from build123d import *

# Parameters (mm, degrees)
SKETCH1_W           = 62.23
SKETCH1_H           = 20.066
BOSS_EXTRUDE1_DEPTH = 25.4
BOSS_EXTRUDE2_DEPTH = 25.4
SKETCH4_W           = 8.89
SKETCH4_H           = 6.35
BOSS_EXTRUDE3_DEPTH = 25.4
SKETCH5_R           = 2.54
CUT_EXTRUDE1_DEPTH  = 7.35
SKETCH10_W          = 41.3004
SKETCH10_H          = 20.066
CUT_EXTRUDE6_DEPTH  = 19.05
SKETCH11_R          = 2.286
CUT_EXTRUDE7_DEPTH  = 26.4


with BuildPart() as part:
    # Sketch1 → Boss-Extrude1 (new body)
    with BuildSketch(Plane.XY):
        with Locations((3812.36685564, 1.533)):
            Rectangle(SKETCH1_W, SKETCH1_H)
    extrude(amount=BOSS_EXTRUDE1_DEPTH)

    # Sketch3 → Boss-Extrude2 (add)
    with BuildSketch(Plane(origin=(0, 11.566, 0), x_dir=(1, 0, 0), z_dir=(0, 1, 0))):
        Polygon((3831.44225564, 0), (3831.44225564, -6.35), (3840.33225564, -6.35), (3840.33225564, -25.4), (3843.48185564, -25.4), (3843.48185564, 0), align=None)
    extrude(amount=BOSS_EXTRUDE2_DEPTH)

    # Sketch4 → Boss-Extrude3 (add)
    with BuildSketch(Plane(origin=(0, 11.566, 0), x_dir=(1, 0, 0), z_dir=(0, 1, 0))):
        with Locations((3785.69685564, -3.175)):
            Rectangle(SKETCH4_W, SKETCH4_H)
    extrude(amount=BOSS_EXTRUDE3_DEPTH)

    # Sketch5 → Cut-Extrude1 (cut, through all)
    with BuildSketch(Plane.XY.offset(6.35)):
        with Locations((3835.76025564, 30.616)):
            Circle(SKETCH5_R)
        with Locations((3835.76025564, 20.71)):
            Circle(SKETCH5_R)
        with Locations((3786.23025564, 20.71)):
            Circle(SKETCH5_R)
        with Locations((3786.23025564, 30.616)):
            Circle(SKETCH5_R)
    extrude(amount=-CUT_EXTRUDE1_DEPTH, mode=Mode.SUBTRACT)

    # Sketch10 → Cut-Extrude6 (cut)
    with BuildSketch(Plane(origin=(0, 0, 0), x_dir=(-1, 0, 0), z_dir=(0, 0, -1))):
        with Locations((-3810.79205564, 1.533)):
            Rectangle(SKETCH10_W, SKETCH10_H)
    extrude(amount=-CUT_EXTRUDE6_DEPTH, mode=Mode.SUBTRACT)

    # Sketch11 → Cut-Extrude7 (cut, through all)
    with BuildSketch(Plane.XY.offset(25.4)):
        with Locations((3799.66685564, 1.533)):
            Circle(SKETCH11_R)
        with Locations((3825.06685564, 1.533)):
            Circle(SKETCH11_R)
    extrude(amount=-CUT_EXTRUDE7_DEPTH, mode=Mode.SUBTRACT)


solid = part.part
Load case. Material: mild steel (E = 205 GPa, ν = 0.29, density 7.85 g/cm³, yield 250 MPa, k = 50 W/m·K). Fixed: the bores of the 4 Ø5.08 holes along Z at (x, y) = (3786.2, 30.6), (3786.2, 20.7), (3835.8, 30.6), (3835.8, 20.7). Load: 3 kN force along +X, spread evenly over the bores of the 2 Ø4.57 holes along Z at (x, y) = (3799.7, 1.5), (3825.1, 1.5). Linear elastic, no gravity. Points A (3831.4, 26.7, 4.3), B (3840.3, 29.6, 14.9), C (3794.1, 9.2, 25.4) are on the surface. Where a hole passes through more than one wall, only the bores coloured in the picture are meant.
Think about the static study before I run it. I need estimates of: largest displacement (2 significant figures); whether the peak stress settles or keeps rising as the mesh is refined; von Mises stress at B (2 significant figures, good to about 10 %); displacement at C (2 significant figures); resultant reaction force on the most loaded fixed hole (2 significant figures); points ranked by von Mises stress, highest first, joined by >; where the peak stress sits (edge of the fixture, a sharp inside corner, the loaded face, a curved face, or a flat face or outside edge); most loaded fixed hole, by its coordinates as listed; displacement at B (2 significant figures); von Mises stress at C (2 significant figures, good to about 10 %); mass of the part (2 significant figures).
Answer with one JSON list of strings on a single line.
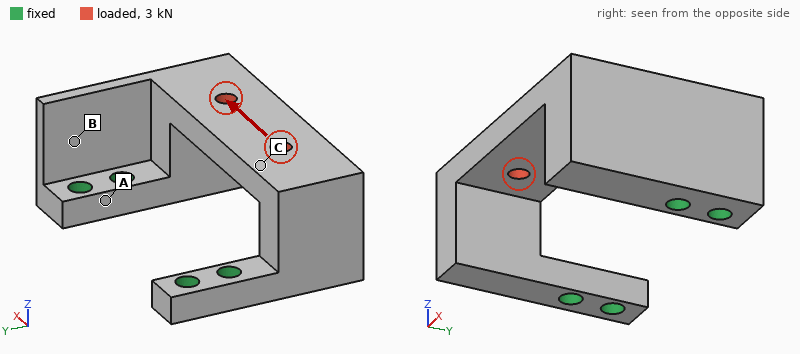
["55 µm", "keeps rising", "42 MPa", "47 µm", "2.5 kN", "C > B > A", "edge of the fixture", "(3835.8, 20.7)", "9.6 µm", "72 MPa", "160 g"]
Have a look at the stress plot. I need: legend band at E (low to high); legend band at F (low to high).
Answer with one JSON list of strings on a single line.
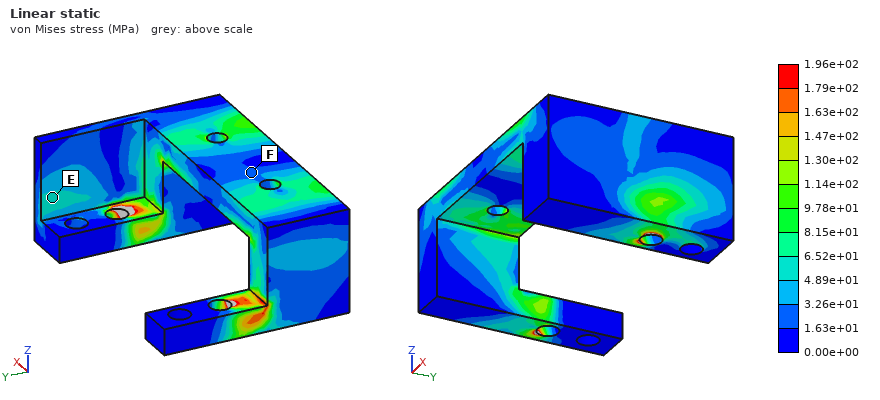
["4.89e+01 to 6.52e+01 MPa", "1.63e+01 to 3.26e+01 MPa"]
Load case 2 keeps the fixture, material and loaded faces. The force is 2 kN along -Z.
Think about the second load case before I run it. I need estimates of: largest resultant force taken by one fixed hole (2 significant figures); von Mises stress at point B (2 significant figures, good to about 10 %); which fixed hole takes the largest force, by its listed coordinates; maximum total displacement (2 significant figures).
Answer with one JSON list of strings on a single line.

["2.1 kN", "24 MPa", "(3835.8, 20.7)", "63 µm"]
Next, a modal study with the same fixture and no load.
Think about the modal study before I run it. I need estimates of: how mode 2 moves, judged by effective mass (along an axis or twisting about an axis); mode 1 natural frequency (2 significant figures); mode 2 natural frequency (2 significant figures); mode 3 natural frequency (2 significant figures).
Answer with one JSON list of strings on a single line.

["along X", "2800 Hz", "4500 Hz", "5600 Hz"]
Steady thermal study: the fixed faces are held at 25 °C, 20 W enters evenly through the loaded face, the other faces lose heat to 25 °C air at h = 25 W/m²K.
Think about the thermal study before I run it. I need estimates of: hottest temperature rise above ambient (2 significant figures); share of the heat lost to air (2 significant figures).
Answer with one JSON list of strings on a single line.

["55 K", "26 %"]
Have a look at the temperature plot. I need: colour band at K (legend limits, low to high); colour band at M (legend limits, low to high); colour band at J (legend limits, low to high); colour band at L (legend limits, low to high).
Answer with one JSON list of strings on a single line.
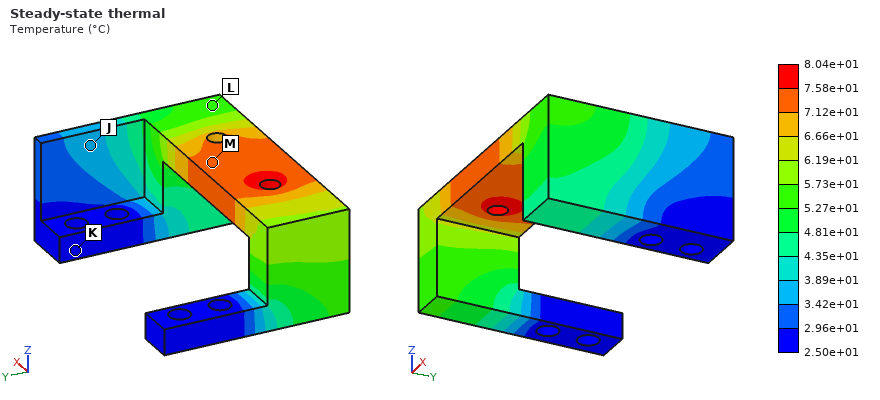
["2.50e+01 to 2.96e+01 °C", "7.12e+01 to 7.58e+01 °C", "3.42e+01 to 3.89e+01 °C", "5.27e+01 to 5.73e+01 °C"]
